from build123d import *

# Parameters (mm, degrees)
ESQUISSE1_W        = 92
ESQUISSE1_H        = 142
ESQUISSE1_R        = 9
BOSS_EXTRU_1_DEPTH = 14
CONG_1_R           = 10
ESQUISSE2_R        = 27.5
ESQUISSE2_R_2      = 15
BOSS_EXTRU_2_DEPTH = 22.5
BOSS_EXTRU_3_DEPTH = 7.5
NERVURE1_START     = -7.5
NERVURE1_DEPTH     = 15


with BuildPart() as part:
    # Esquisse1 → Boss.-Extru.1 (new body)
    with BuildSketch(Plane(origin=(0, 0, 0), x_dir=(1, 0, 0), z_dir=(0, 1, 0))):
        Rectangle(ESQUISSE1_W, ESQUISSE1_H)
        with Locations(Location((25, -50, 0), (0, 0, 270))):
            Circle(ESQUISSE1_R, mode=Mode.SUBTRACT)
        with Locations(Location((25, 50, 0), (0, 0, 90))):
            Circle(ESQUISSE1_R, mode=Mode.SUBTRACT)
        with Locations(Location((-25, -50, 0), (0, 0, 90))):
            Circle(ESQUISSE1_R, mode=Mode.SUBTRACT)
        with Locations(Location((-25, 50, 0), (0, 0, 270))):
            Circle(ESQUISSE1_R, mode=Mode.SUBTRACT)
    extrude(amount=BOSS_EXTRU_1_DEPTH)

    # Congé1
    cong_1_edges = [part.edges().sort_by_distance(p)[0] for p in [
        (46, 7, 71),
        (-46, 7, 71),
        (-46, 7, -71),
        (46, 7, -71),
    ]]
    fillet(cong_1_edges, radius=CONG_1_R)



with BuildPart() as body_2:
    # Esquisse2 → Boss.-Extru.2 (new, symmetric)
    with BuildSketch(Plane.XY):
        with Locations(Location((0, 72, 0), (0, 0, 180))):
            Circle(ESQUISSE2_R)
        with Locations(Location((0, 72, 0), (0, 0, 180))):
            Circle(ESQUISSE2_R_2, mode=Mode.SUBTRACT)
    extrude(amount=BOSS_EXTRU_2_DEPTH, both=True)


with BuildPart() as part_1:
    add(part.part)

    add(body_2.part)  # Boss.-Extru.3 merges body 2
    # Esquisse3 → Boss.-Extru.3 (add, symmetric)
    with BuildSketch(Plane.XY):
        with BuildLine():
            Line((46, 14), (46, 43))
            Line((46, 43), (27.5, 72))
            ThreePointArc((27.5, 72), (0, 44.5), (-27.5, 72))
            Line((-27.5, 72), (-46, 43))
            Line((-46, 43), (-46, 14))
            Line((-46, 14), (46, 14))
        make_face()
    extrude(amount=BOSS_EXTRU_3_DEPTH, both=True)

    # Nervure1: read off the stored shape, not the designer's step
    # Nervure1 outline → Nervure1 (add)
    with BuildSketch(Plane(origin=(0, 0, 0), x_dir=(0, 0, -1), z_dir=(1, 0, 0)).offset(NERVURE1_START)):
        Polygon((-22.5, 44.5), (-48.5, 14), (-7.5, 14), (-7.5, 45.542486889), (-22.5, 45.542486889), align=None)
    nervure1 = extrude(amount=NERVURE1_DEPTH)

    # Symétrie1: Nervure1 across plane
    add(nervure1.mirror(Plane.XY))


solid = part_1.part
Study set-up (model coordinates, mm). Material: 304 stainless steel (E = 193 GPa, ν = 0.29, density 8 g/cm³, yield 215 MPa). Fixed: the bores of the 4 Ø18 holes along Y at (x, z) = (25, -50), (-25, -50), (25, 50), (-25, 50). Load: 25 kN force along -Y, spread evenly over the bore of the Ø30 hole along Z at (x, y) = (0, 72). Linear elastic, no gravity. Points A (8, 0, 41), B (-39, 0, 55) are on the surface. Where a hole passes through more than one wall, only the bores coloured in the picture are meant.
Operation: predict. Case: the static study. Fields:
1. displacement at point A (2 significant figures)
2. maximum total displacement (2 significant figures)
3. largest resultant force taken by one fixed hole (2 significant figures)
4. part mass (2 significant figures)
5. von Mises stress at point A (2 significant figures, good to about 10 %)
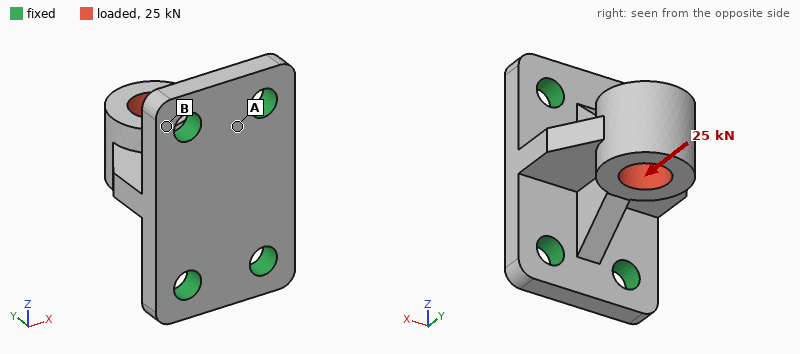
4.0 µm
20 µm
6.8 kN
2.6 kg
17 MPa
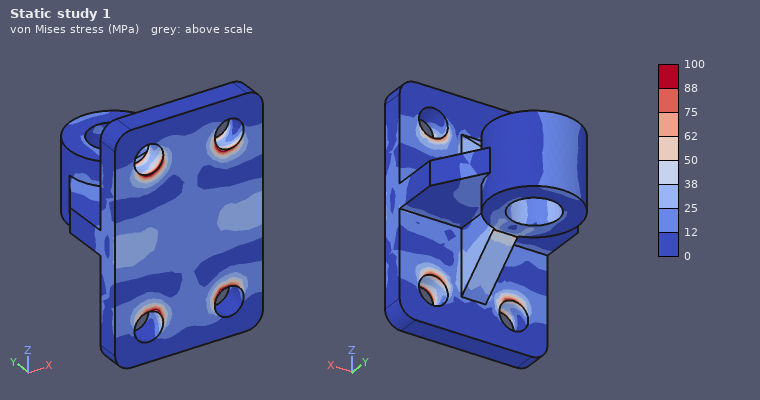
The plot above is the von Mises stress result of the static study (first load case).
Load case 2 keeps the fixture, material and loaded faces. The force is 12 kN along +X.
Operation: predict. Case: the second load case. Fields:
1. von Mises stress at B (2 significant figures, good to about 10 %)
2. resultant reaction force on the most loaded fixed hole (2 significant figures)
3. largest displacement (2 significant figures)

20 MPa
8.0 kN
84 µm
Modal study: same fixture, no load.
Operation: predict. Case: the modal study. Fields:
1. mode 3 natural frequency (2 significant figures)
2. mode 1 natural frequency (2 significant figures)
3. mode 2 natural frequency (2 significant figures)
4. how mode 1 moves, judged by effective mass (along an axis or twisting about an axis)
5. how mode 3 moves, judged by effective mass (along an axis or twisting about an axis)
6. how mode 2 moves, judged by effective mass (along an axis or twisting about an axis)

5400 Hz
2400 Hz
3500 Hz
along X
along Y
along Z
